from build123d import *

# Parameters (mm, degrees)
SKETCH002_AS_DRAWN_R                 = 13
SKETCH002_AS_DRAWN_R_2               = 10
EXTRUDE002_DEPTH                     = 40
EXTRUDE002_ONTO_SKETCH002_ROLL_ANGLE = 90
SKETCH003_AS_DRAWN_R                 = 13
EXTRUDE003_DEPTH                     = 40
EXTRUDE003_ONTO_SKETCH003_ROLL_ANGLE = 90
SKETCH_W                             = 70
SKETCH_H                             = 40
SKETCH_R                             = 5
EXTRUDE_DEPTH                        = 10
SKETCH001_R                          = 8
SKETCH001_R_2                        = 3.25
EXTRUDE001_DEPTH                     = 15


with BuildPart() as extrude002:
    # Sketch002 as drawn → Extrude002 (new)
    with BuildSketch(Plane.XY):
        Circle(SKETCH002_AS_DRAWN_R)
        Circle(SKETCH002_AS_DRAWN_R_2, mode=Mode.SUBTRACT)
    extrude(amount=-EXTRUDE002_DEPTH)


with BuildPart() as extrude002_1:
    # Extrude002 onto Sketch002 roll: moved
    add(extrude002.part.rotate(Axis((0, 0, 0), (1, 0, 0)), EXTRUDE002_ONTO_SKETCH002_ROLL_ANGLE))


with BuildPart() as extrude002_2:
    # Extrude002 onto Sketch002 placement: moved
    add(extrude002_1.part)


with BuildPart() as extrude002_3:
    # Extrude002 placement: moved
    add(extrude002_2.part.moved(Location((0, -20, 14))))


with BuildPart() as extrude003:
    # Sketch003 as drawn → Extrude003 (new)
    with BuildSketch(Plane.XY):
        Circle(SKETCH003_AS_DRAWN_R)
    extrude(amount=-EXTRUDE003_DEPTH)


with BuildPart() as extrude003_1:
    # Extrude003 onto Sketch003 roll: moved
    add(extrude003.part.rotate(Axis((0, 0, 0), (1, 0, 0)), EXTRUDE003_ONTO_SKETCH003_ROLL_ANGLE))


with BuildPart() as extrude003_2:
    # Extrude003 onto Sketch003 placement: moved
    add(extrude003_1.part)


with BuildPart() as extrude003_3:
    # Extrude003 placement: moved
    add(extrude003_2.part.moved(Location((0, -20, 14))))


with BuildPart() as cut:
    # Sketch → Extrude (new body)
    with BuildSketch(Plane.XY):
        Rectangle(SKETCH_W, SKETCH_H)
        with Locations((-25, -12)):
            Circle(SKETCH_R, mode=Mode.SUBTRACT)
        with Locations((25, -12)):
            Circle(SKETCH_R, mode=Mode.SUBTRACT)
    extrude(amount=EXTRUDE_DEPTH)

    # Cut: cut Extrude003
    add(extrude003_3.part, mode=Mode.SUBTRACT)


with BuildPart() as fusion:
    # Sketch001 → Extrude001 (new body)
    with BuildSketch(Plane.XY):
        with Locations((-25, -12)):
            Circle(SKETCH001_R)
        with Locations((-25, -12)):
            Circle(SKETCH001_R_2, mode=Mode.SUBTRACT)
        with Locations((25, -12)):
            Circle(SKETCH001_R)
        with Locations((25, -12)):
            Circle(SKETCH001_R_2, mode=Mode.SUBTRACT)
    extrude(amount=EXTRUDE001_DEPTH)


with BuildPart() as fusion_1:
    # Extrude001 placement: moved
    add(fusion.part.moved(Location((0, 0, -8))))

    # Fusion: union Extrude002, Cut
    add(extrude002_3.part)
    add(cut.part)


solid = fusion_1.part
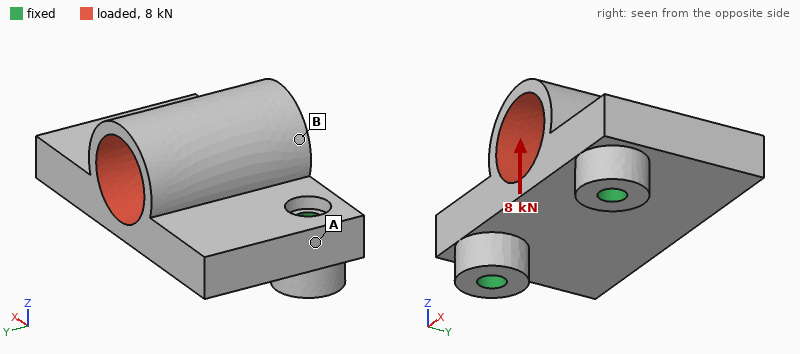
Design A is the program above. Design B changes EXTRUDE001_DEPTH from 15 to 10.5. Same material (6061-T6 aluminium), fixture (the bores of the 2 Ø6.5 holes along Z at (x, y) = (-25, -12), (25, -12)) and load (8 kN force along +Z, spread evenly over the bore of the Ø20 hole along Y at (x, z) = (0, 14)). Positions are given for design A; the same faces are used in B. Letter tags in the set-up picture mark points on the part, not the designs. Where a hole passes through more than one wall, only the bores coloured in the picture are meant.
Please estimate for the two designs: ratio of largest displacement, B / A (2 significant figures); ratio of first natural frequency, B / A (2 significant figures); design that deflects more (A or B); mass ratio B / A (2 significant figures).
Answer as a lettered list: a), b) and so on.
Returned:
a) 1.5
b) 0.77
c) B
d) 0.99
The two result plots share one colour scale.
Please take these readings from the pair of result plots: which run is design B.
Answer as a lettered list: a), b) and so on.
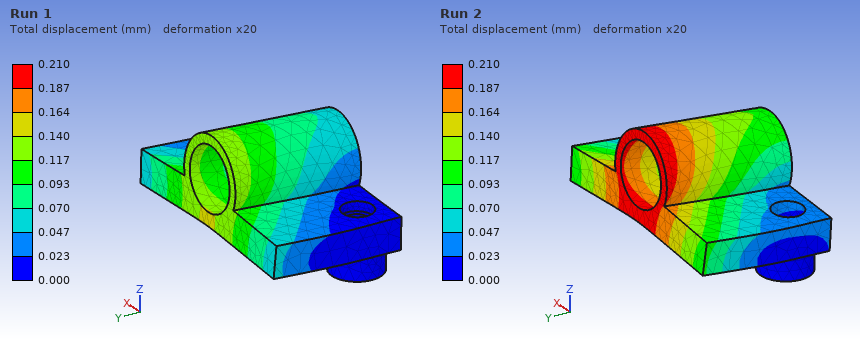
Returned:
a) Run 2
